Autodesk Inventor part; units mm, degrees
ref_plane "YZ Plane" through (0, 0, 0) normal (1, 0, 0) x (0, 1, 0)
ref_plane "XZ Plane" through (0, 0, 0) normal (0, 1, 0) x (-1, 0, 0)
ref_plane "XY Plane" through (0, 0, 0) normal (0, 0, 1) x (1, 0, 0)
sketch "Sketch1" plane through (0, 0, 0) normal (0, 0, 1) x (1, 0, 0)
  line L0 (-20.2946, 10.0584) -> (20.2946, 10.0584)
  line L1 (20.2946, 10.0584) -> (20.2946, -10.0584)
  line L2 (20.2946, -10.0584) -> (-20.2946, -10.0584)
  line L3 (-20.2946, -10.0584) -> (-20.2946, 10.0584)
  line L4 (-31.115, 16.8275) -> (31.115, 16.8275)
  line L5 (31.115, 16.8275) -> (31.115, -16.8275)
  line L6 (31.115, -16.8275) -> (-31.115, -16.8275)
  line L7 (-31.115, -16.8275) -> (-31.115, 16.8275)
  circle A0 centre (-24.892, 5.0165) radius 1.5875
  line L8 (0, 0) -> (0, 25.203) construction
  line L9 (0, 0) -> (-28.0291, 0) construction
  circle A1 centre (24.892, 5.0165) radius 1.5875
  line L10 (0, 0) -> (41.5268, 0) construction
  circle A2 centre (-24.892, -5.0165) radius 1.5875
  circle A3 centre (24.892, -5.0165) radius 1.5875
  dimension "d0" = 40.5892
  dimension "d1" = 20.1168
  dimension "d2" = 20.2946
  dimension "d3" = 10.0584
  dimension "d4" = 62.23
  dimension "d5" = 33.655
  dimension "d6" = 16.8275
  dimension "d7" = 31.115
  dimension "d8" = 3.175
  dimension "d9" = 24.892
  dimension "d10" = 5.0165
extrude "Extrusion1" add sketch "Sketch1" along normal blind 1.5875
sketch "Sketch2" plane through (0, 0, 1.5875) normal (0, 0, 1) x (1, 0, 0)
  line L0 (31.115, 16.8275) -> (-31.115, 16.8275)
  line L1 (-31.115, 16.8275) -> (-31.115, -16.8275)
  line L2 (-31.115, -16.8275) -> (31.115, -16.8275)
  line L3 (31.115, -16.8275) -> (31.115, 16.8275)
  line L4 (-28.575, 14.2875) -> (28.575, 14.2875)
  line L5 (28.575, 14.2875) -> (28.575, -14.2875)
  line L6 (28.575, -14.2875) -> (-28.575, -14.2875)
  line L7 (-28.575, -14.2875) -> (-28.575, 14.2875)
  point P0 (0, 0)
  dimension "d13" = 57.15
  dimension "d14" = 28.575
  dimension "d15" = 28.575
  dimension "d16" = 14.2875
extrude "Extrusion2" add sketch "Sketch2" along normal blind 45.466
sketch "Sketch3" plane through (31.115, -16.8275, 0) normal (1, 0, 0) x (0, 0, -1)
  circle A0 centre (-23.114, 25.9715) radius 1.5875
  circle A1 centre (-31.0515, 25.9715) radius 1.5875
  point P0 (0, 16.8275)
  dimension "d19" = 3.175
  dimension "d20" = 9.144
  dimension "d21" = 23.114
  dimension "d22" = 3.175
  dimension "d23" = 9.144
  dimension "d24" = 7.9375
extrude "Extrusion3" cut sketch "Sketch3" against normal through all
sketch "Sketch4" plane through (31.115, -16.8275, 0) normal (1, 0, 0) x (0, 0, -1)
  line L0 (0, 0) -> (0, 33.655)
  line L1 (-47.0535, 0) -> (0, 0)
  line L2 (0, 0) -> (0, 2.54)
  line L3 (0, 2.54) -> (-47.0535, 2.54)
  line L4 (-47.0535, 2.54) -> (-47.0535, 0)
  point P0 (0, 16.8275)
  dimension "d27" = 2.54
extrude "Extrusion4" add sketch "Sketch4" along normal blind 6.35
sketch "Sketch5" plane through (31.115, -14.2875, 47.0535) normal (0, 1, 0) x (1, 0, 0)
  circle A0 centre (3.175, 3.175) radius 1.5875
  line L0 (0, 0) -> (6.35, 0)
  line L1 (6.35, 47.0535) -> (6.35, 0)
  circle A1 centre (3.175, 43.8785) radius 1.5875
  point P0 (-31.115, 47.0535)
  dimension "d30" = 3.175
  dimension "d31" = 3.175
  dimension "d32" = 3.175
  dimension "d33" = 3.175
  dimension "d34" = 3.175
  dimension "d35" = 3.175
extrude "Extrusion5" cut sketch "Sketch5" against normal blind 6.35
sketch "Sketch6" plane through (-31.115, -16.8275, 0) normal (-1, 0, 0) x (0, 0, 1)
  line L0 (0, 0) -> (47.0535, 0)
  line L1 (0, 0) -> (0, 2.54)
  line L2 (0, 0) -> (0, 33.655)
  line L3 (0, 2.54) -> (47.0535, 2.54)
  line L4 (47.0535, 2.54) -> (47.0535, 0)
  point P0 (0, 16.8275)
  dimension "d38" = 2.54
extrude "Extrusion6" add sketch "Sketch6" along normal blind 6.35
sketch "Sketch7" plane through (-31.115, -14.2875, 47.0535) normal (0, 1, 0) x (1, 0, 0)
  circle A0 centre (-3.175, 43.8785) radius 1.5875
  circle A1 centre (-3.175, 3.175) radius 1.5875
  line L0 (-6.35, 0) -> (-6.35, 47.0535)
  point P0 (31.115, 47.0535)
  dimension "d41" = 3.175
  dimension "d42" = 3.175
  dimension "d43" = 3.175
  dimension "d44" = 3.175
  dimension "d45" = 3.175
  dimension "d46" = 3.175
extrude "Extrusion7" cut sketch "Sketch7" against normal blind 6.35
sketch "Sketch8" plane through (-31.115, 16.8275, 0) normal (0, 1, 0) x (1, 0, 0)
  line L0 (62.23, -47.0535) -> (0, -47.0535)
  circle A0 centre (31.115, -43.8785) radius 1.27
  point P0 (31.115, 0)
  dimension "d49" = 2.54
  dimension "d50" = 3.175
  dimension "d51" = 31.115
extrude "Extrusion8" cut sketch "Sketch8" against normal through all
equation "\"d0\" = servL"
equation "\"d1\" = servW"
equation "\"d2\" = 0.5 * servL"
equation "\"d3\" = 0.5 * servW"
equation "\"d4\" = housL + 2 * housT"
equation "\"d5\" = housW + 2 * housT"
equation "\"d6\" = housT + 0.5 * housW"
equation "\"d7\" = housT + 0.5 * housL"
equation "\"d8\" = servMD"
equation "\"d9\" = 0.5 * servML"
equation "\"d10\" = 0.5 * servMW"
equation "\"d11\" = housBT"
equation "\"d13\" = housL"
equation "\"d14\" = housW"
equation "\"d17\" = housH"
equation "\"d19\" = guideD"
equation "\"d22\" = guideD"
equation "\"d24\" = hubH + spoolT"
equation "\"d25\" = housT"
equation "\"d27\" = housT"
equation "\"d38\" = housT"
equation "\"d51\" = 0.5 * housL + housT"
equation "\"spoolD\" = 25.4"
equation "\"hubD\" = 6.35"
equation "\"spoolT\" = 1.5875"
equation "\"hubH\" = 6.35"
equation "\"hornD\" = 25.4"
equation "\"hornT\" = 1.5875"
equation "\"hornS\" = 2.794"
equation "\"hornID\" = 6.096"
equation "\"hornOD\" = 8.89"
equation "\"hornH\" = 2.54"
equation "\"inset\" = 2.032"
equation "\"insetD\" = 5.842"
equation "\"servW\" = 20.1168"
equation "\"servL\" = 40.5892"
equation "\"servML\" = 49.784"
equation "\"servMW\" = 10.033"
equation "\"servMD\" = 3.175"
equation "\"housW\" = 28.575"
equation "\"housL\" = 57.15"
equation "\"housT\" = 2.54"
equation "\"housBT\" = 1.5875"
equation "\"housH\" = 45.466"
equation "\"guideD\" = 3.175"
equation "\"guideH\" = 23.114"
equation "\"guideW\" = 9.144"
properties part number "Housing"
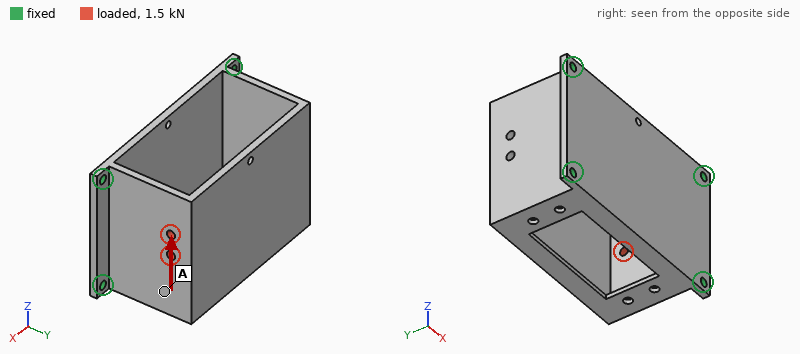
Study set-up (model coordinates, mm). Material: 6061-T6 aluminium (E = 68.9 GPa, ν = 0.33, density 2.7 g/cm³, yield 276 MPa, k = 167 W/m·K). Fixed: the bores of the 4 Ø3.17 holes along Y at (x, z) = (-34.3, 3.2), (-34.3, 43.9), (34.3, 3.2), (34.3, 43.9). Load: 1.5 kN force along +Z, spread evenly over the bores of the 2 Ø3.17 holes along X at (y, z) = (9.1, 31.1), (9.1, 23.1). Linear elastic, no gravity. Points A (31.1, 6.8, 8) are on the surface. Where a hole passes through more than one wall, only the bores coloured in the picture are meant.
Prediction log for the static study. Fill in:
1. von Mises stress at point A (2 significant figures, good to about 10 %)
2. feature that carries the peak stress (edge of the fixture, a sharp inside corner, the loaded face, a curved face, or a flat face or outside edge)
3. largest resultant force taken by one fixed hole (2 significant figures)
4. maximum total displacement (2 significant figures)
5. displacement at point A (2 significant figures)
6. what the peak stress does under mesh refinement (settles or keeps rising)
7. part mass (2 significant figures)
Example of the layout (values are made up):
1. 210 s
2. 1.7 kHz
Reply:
1. 15 MPa
2. edge of the fixture
3. 1.2 kN
4. 64 µm
5. 37 µm
6. keeps rising
7. 66 g
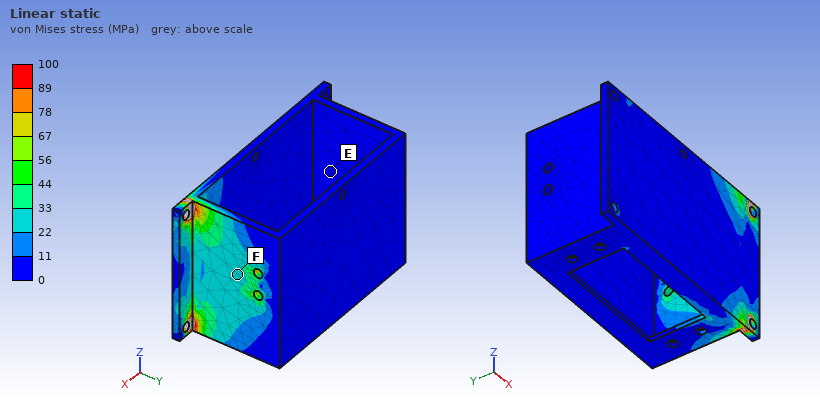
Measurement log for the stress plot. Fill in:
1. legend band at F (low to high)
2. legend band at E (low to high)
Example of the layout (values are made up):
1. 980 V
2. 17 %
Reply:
1. 22 to 33 MPa
2. 0 to 11 MPa
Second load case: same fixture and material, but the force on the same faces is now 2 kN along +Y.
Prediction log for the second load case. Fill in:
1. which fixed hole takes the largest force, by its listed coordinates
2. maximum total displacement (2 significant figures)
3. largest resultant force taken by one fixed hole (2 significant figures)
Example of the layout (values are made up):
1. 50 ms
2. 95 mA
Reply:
1. (34.3, 43.9)
2. 56 µm
3. 1.2 kN
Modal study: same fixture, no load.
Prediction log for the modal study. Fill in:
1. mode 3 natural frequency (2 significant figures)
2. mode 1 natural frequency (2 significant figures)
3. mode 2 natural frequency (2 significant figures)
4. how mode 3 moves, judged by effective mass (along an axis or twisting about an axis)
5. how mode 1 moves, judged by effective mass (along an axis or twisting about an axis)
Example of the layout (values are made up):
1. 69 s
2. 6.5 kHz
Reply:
1. 3300 Hz
2. 2200 Hz
3. 3100 Hz
4. along Y
5. along X
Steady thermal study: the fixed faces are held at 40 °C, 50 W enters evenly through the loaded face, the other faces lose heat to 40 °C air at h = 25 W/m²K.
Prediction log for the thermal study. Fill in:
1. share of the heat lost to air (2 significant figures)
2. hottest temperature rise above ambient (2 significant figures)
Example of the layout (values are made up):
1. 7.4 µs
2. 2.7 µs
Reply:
1. 22 %
2. 74 K
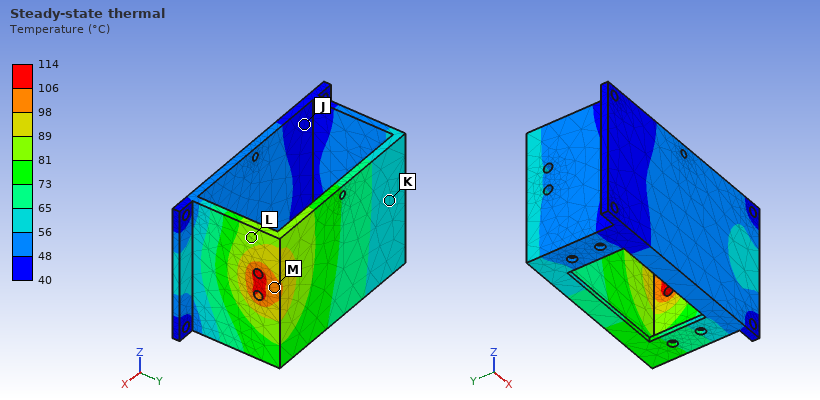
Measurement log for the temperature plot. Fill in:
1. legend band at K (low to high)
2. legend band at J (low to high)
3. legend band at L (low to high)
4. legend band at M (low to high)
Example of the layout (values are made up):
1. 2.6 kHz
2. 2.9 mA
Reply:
1. 56 to 65 °C
2. 40 to 48 °C
3. 81 to 89 °C
4. 98 to 106 °C
